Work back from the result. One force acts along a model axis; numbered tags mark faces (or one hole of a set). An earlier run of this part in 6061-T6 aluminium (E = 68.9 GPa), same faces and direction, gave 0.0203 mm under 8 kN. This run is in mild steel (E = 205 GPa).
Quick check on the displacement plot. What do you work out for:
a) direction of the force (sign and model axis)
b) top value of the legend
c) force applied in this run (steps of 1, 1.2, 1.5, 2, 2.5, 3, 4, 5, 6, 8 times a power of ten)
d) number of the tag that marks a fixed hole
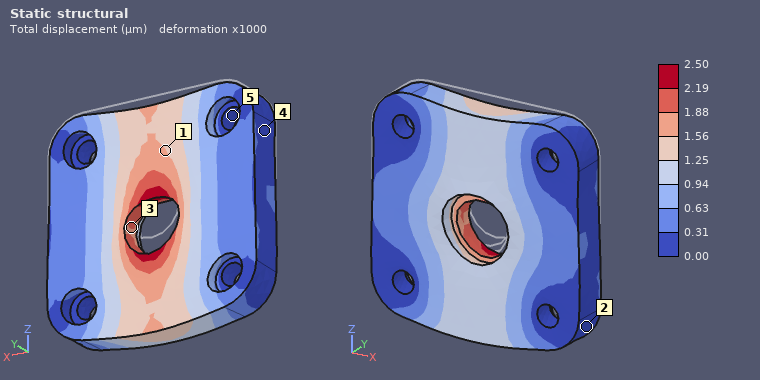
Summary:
-Z
2.50 µm
3 kN
5
